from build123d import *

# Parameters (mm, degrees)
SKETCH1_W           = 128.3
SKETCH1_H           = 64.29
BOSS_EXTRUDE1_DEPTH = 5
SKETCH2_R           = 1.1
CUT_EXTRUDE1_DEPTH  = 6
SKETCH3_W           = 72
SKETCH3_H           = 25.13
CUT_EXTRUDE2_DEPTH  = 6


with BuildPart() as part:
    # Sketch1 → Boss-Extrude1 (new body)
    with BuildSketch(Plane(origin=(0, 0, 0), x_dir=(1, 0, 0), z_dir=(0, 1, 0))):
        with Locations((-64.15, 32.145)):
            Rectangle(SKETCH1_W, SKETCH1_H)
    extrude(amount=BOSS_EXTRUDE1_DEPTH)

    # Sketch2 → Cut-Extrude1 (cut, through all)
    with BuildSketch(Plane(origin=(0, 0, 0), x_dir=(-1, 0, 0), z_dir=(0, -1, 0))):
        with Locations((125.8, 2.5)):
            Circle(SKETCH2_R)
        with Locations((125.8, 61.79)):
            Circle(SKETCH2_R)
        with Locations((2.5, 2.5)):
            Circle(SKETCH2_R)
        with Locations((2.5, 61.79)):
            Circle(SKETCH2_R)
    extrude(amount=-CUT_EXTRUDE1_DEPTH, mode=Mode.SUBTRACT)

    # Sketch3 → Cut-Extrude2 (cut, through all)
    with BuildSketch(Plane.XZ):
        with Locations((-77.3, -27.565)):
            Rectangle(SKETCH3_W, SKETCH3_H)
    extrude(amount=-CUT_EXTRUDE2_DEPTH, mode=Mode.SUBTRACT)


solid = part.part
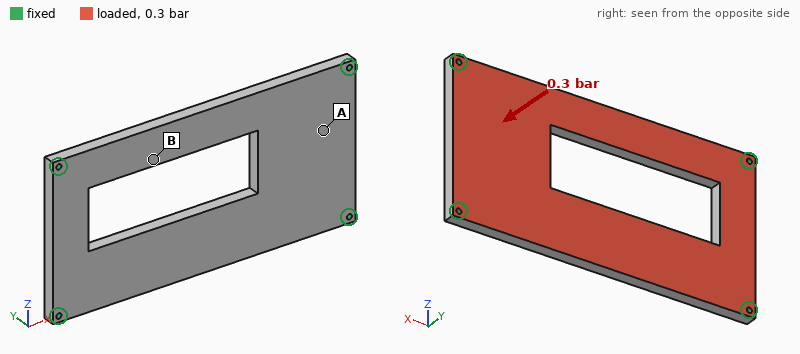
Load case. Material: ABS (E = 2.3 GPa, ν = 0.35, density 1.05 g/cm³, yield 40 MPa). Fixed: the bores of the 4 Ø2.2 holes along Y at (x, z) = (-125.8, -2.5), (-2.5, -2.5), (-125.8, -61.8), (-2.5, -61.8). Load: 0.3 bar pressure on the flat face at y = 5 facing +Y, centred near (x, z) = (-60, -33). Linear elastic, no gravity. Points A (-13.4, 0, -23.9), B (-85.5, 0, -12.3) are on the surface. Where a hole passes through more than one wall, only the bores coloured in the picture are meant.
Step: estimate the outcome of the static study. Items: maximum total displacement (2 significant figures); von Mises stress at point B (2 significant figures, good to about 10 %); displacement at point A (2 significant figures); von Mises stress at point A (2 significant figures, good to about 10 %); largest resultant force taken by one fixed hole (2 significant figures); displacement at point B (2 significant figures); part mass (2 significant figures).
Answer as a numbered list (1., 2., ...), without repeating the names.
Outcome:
1. 1.4 mm
2. 3.9 MPa
3. 0.33 mm
4. 2.3 MPa
5. 53 N
6. 1.00 mm
7. 34 g
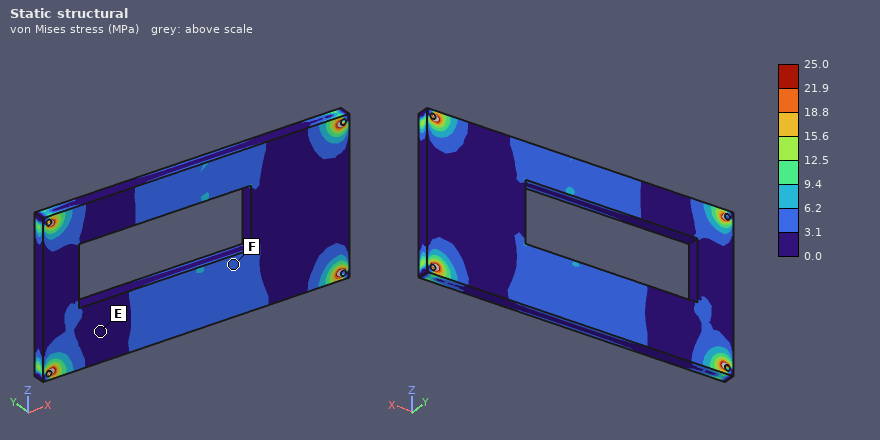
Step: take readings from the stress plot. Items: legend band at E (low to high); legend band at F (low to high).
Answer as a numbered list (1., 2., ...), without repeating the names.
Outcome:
1. 0.0 to 3.1 MPa
2. 3.1 to 6.2 MPa
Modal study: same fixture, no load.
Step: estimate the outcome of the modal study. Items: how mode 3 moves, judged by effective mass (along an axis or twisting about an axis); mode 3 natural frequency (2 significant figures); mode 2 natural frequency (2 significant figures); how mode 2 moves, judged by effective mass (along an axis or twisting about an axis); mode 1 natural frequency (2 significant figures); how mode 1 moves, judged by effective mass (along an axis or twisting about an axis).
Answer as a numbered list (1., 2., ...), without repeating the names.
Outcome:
1. twisting about Z
2. 1000 Hz
3. 610 Hz
4. twisting about X
5. 390 Hz
6. along Y
